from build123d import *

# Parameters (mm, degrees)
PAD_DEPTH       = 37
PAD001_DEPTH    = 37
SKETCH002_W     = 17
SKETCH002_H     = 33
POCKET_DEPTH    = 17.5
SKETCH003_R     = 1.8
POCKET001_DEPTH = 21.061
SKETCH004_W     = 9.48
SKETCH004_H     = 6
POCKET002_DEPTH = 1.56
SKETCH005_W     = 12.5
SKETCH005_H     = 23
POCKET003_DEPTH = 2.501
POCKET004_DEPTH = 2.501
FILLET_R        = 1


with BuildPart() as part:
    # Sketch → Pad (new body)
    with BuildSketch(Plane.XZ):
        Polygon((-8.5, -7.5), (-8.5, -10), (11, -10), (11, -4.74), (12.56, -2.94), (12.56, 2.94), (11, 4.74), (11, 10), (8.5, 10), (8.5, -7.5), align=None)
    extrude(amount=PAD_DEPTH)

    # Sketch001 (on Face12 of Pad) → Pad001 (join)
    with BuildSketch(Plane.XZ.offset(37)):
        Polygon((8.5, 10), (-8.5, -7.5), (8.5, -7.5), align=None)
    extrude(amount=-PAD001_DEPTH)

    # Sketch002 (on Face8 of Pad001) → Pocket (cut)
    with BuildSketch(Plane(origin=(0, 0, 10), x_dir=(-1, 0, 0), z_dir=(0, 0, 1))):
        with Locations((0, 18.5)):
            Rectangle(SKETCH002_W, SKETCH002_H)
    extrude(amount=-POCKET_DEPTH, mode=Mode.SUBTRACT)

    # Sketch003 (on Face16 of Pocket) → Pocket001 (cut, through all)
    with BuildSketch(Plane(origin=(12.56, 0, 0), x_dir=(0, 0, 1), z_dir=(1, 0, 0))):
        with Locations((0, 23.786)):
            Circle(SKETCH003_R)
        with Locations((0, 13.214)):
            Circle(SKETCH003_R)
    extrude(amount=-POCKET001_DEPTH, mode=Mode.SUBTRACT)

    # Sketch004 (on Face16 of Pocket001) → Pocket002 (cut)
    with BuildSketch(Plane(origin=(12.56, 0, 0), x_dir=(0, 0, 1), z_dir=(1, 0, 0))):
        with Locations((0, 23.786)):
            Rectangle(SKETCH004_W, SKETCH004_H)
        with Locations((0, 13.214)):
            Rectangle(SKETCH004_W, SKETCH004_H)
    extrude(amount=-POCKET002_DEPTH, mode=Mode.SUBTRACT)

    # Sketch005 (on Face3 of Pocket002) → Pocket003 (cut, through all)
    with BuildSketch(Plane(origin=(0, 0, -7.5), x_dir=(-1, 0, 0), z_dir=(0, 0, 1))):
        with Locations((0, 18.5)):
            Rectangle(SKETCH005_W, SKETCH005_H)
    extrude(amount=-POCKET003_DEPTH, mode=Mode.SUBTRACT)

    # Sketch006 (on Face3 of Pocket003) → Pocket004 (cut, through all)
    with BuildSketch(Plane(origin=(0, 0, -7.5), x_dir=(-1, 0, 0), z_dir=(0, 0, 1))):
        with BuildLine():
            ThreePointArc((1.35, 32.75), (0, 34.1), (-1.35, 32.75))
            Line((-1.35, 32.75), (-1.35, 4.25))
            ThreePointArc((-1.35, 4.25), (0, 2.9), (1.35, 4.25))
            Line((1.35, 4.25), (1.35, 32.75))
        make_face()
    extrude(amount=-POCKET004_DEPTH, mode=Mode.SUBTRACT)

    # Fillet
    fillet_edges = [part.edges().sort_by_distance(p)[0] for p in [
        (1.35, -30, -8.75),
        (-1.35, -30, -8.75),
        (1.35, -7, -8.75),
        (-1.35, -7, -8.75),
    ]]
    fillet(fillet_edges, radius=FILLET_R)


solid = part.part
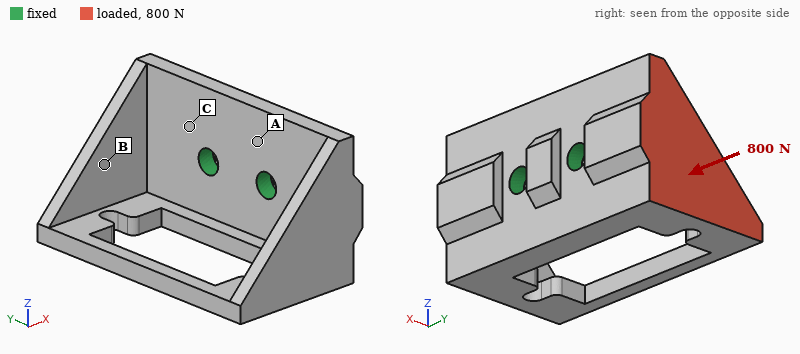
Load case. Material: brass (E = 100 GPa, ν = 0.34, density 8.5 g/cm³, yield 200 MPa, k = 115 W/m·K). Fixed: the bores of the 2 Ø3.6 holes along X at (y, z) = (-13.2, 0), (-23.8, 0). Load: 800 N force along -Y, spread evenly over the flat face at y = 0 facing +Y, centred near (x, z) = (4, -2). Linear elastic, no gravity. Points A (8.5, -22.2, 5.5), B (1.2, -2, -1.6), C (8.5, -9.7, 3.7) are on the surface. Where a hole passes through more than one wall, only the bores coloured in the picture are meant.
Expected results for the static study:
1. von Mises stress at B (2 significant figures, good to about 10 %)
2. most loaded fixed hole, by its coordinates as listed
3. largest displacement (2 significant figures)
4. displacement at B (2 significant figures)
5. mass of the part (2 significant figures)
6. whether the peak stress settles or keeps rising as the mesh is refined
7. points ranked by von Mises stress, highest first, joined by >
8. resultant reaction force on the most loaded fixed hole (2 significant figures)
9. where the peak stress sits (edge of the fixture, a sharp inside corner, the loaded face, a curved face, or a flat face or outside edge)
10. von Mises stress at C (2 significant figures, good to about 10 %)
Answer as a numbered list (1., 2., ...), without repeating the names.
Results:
1. 50 MPa
2. (-13.2, 0)
3. 0.11 mm
4. 0.069 mm
5. 30 g
6. keeps rising
7. C > B > A
8. 580 N
9. edge of the fixture
10. 83 MPa
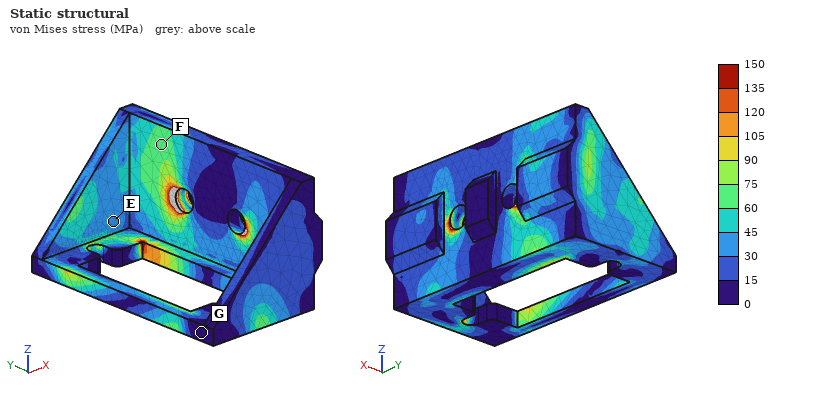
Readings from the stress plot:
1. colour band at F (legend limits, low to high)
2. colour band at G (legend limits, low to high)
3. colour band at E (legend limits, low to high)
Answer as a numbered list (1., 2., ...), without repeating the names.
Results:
1. 60 to 75 MPa
2. 0 to 15 MPa
3. 30 to 45 MPa
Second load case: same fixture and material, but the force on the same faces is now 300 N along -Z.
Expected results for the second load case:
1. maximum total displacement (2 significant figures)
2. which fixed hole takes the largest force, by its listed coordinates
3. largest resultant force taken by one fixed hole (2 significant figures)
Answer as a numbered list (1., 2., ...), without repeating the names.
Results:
1. 63 µm
2. (-13.2, 0)
3. 550 N
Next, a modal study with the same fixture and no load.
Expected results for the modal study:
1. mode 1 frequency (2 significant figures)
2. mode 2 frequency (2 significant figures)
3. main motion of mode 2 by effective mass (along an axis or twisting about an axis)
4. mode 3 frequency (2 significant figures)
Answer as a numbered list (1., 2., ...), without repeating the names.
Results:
1. 3300 Hz
2. 3700 Hz
3. along Z
4. 5300 Hz
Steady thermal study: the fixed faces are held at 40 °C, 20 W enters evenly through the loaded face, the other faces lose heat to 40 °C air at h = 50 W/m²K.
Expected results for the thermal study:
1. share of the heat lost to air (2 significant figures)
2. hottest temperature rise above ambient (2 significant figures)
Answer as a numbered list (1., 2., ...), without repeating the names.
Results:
1. 10 %
2. 51 K
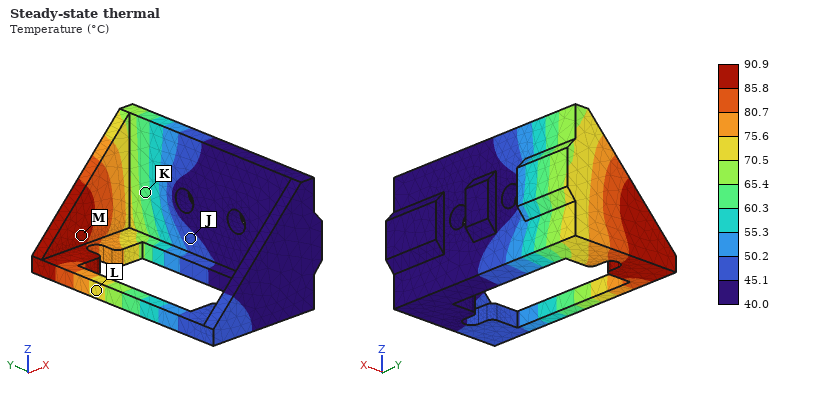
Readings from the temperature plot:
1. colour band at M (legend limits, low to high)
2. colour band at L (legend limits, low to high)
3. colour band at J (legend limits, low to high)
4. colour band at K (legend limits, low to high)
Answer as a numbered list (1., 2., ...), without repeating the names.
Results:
1. 85.8 to 90.9 °C
2. 70.5 to 75.6 °C
3. 45.1 to 50.2 °C
4. 60.3 to 65.4 °C
